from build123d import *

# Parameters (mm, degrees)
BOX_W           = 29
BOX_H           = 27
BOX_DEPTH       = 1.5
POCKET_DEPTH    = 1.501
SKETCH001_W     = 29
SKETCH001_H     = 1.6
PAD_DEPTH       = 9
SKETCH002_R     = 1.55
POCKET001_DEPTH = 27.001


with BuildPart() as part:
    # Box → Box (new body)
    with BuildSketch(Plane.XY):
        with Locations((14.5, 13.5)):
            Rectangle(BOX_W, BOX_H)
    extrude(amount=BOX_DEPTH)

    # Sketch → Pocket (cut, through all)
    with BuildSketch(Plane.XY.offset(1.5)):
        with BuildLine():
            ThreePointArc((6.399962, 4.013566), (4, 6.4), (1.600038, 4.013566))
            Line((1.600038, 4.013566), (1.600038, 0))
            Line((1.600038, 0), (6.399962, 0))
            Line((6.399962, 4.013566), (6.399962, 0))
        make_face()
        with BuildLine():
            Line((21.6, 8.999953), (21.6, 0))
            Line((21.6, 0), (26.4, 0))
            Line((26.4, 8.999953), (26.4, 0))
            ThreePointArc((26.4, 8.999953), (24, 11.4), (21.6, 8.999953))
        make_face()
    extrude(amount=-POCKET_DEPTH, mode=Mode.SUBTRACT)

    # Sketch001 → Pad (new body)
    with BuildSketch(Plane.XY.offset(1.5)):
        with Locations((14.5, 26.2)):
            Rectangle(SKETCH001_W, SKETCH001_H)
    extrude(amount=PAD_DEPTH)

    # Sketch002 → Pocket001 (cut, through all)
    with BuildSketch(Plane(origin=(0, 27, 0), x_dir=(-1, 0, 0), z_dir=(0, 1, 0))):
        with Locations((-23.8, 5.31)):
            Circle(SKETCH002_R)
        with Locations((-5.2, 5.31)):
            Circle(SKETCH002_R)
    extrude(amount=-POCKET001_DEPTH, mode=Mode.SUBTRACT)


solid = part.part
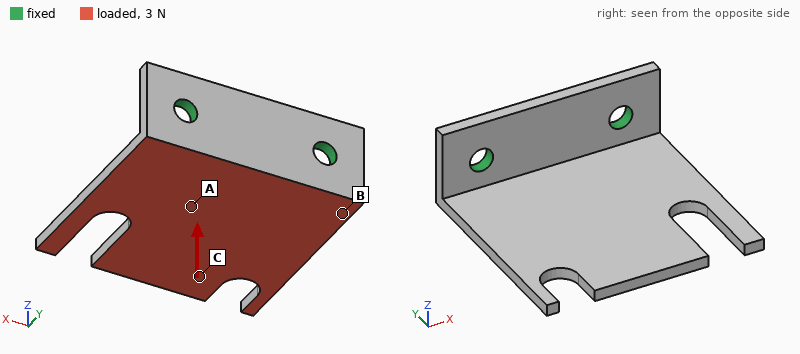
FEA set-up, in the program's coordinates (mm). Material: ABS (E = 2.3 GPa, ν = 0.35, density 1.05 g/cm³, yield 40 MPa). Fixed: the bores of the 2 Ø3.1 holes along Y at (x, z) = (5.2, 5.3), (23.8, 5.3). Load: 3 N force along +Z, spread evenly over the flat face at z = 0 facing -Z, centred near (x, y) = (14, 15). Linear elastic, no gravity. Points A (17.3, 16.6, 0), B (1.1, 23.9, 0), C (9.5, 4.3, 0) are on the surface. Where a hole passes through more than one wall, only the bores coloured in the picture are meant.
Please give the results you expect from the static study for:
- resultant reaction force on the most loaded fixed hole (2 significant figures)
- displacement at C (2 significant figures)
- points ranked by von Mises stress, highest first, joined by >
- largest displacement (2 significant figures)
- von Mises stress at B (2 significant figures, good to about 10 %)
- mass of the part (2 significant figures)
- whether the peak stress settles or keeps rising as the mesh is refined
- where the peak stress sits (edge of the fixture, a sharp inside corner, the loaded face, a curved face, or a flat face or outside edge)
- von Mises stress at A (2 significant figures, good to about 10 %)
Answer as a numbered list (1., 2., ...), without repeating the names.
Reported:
1. 1.6 N
2. 0.34 mm
3. B > A > C
4. 0.43 mm
5. 2.5 MPa
6. 1.5 g
7. keeps rising
8. edge of the fixture
9. 1.1 MPa
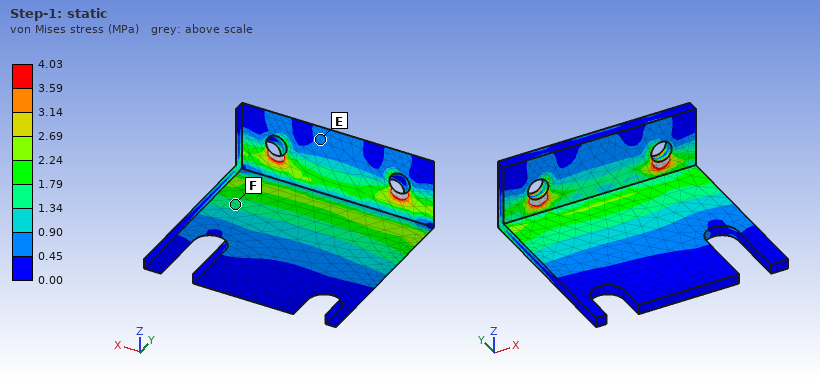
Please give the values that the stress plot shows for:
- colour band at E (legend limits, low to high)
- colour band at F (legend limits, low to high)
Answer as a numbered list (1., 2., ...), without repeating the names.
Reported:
1. 0.45 to 0.90 MPa
2. 1.34 to 1.79 MPa
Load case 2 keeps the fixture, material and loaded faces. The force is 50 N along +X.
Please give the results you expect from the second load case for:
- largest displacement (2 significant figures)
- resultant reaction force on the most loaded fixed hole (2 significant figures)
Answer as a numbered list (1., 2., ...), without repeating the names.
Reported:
1. 0.29 mm
2. 40 N
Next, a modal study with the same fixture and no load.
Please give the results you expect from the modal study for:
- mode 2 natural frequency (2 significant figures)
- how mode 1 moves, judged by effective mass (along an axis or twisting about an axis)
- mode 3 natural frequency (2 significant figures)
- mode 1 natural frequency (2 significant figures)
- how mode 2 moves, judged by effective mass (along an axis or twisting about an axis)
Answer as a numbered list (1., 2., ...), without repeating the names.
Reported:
1. 1100 Hz
2. along Z
3. 2000 Hz
4. 510 Hz
5. twisting about Y
